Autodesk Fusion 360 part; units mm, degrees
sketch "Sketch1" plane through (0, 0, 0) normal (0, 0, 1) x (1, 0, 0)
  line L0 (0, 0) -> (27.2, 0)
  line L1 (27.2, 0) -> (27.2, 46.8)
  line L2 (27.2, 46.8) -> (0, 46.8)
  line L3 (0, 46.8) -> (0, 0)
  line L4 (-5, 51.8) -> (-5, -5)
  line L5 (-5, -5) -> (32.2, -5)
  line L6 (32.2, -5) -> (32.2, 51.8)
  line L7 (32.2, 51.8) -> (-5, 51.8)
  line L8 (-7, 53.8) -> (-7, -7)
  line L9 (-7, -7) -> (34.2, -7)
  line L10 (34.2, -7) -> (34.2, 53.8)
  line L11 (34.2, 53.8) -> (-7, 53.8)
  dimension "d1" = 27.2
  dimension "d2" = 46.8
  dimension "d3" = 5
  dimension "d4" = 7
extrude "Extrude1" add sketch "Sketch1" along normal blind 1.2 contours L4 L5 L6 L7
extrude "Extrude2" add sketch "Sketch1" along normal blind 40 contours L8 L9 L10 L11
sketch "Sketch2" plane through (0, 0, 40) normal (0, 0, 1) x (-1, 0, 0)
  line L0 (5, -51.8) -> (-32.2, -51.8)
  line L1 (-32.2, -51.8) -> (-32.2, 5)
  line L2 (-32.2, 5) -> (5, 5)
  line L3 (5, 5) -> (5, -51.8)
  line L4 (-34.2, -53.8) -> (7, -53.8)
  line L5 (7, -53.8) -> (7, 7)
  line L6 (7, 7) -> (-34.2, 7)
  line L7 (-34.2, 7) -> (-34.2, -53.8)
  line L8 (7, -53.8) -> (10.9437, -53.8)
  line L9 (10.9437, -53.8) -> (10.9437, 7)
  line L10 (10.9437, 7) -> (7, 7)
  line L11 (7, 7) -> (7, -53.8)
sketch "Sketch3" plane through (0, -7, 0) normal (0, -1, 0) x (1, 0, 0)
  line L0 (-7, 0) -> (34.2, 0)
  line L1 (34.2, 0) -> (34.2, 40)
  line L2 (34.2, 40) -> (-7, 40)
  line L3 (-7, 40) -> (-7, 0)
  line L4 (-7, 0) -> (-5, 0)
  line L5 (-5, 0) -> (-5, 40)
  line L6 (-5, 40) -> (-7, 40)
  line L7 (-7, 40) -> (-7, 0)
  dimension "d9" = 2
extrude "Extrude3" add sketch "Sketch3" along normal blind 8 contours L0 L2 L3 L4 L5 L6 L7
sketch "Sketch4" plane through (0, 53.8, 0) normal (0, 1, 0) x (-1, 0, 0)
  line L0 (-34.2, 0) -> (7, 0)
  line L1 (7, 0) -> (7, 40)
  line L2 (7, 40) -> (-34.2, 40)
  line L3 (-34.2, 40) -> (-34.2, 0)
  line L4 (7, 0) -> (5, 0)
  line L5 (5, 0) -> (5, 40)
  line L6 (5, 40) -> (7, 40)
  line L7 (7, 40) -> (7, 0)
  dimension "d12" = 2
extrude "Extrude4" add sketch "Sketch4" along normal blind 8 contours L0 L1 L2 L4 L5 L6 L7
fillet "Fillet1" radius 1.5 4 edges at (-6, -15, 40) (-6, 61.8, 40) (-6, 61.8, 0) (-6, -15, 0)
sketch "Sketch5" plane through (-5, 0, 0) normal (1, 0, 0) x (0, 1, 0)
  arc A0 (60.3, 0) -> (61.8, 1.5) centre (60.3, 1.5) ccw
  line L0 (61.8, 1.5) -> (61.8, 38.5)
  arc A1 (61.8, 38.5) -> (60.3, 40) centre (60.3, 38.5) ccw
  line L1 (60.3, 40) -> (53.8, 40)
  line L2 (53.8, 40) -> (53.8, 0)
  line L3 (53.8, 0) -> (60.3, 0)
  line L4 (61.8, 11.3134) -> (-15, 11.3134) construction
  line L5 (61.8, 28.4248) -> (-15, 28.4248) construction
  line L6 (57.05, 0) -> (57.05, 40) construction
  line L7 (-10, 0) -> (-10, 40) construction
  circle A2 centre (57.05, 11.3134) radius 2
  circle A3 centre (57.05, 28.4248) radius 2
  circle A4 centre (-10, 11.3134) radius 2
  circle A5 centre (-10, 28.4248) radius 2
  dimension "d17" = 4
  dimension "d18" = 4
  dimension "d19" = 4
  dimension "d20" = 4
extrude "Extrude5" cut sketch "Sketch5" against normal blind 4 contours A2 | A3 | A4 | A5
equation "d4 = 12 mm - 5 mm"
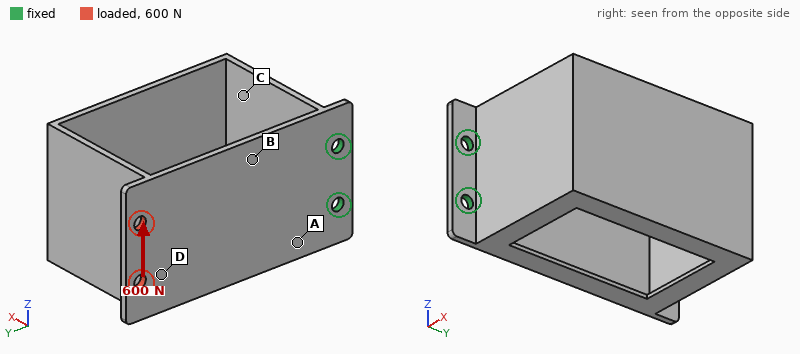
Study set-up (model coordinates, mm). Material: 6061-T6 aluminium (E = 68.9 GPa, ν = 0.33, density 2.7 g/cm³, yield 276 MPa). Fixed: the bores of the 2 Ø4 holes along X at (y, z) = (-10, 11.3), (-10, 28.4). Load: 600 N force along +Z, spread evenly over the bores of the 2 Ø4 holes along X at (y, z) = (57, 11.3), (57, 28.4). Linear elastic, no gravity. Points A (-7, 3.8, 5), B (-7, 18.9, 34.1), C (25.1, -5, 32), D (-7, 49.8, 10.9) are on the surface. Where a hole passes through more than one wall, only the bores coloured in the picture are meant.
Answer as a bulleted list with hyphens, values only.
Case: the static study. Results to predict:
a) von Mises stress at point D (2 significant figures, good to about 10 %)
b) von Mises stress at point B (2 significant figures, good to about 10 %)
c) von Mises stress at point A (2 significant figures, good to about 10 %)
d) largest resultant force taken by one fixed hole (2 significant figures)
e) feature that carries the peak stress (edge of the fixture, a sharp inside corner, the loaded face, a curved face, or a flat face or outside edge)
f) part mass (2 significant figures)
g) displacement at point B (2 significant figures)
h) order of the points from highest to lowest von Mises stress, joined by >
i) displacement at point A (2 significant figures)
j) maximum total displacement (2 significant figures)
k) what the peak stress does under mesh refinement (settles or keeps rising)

- 16 MPa
- 29 MPa
- 43 MPa
- 2.0 kN
- edge of the fixture
- 48 g
- 0.064 mm
- A > B > D > C
- 0.033 mm
- 0.18 mm
- keeps rising
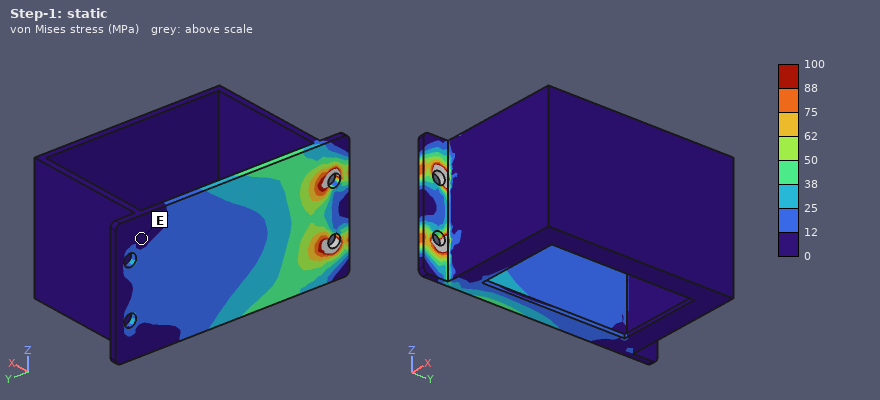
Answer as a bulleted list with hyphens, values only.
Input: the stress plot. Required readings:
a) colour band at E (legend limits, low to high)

- 0 to 12 MPa
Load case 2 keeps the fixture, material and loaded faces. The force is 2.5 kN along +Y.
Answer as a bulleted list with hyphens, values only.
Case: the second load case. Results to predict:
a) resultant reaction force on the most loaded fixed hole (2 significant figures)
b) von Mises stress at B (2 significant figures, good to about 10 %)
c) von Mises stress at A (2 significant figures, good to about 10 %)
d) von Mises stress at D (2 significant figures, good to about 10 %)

- 1.3 kN
- 33 MPa
- 27 MPa
- 44 MPa
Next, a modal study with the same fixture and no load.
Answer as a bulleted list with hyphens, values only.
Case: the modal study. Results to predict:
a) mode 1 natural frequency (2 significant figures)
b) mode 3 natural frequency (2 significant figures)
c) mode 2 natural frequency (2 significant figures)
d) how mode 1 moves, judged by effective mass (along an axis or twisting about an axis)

- 250 Hz
- 1600 Hz
- 710 Hz
- along X
